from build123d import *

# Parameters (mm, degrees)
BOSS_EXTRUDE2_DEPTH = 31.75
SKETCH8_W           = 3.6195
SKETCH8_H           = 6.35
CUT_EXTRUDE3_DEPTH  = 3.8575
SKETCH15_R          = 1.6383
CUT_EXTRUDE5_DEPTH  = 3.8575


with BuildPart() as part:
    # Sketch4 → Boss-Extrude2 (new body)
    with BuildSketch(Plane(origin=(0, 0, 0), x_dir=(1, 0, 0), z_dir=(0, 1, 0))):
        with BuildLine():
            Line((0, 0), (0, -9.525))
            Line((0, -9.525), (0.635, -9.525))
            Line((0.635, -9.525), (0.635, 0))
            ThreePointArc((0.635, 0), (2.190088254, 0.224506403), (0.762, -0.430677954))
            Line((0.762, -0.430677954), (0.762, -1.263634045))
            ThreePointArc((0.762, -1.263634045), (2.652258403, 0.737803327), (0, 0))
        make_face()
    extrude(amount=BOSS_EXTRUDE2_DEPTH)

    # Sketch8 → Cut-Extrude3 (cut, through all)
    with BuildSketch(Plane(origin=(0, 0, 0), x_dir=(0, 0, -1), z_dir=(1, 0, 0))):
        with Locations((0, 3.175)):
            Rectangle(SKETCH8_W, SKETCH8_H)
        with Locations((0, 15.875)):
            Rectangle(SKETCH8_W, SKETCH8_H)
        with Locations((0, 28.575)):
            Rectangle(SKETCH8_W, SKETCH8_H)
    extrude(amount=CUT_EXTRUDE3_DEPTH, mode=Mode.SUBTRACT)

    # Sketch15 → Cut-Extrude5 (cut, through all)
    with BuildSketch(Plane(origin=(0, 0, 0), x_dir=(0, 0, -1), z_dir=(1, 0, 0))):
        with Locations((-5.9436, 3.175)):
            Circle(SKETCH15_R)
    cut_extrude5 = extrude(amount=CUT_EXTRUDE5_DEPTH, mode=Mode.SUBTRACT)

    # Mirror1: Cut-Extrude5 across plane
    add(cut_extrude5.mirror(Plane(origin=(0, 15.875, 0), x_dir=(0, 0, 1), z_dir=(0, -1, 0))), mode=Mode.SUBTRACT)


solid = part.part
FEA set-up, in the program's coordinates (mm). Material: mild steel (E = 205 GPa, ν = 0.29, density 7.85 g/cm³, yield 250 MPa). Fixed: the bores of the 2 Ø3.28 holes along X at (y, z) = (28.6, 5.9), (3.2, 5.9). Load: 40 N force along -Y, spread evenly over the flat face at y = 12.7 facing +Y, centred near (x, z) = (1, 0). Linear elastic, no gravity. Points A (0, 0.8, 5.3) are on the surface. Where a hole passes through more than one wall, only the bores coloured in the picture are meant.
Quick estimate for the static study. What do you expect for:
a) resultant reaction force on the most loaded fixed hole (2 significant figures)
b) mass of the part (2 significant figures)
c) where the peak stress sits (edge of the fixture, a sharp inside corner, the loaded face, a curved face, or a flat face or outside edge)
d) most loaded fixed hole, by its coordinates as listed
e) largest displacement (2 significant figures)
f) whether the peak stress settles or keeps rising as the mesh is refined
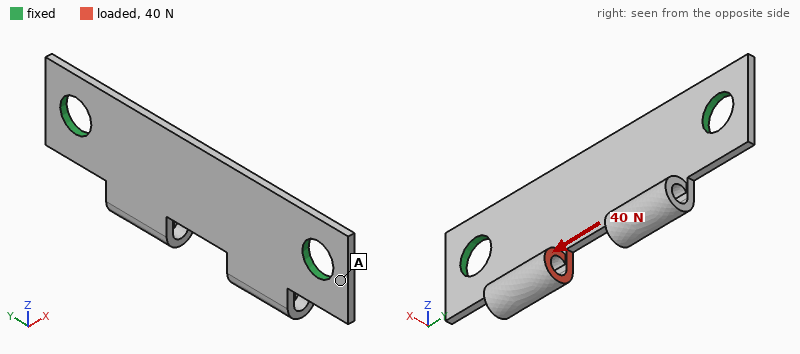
30 N
1.6 g
a sharp inside corner
(3.2, 5.9)
27 µm
keeps rising
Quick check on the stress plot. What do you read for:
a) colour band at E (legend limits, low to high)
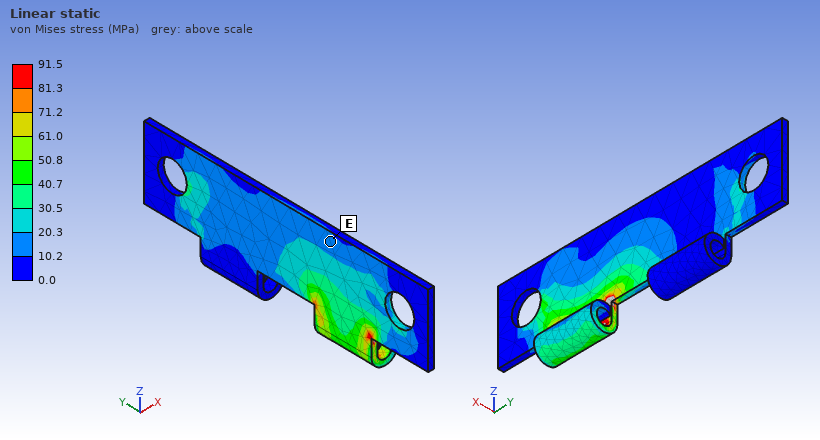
10.2 to 20.3 MPa
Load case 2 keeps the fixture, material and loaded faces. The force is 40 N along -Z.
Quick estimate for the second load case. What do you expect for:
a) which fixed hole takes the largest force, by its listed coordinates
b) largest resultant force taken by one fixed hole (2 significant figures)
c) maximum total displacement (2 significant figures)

(3.2, 5.9)
27 N
42 µm
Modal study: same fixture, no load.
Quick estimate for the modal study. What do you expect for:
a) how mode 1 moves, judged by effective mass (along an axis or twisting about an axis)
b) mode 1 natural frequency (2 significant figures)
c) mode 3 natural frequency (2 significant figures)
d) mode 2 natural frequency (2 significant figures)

along X
4400 Hz
7500 Hz
7400 Hz
